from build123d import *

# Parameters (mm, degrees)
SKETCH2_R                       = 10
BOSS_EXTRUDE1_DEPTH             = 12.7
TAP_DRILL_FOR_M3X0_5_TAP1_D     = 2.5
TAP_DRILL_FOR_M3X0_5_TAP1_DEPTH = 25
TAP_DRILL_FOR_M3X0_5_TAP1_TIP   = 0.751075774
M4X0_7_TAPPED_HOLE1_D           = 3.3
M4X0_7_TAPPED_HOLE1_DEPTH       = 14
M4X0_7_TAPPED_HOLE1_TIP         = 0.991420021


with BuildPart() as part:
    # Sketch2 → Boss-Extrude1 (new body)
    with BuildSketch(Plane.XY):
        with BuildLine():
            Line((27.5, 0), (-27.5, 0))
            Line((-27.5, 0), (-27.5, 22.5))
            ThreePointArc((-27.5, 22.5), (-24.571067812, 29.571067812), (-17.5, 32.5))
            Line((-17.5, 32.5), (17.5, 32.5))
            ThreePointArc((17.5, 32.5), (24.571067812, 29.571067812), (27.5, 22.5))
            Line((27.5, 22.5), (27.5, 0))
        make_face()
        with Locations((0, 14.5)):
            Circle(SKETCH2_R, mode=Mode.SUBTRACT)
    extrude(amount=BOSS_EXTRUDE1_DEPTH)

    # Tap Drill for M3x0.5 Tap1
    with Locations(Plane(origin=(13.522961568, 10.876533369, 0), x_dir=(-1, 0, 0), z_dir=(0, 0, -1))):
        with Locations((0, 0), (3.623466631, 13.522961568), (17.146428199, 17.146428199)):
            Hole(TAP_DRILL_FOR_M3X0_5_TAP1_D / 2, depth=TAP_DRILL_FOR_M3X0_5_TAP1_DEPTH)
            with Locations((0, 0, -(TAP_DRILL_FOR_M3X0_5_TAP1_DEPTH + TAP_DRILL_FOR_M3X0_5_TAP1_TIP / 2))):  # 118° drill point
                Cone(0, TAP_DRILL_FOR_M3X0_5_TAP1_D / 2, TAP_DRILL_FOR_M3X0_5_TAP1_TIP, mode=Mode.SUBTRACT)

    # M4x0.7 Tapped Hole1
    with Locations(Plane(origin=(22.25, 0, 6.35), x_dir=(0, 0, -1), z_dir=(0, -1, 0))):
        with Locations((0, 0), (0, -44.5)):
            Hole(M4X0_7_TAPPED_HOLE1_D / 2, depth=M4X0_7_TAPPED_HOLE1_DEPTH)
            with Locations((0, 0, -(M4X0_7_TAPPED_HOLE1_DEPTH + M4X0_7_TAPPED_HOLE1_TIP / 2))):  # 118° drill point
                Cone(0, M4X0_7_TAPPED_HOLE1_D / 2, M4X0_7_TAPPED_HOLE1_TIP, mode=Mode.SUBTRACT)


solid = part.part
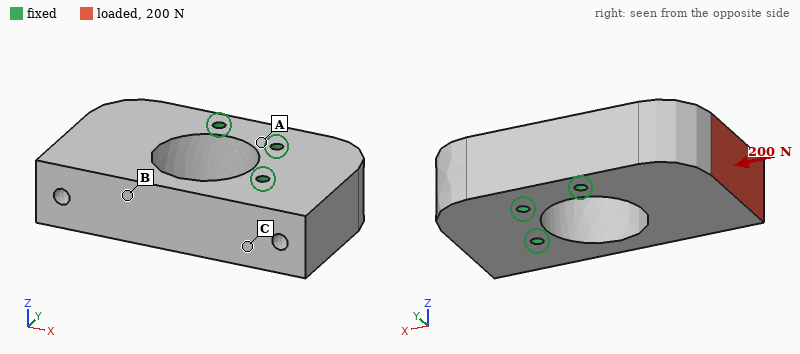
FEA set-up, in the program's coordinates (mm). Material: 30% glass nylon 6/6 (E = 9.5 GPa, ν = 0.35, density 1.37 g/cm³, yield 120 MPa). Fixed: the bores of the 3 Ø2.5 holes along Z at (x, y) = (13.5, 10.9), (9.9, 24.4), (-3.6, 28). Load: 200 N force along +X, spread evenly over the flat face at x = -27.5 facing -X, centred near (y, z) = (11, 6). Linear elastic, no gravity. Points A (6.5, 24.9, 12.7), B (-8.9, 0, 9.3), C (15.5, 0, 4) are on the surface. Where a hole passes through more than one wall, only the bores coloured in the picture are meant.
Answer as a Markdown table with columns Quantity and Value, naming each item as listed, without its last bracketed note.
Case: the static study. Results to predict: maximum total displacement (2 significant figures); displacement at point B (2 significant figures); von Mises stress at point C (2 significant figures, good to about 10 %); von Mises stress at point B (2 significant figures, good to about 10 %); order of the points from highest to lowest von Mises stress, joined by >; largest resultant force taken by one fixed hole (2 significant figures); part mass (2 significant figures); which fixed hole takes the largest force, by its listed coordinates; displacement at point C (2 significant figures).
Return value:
| Quantity | Value |
|---|---|
| maximum total displacement | 13 µm |
| displacement at point B | 8.5 µm |
| von Mises stress at point C | 1.2 MPa |
| von Mises stress at point B | 2.4 MPa |
| order of the points from highest to lowest von Mises stress, joined by > | B > C > A |
| largest resultant force taken by one fixed hole | 160 N |
| part mass | 24 g |
| which fixed hole takes the largest force, by its listed coordinates | (13.5, 10.9) |
| displacement at point C | 3.9 µm |
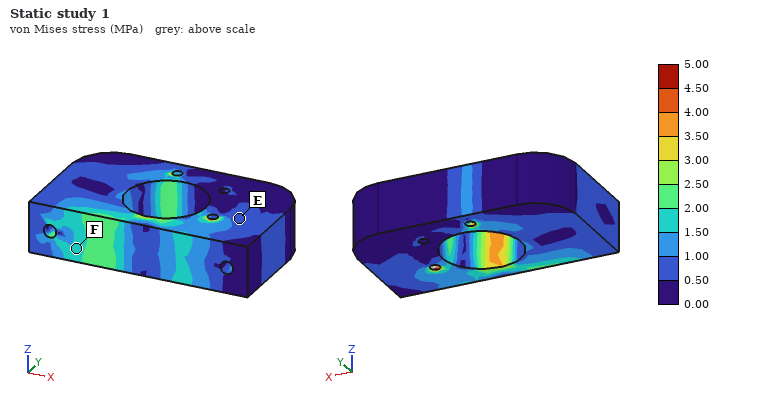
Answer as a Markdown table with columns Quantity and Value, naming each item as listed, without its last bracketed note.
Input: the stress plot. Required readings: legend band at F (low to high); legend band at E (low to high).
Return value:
| Quantity | Value |
|---|---|
| legend band at F | 1.50 to 2.00 MPa |
| legend band at E | 0.50 to 1.00 MPa |
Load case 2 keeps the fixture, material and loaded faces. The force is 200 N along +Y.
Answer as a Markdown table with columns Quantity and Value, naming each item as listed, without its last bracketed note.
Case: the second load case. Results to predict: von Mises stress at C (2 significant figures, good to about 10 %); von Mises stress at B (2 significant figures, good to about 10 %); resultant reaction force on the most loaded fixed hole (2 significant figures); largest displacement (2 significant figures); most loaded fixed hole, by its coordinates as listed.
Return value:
| Quantity | Value |
|---|---|
| von Mises stress at C | 1.8 MPa |
| von Mises stress at B | 2.8 MPa |
| resultant reaction force on the most loaded fixed hole | 290 N |
| largest displacement | 26 µm |
| most loaded fixed hole, by its coordinates as listed | (-3.6, 28) |
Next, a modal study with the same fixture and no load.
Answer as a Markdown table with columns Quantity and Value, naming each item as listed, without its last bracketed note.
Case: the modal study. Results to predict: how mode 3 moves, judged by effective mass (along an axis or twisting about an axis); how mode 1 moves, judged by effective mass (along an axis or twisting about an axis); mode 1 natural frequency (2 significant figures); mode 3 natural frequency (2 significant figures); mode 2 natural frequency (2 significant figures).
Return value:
| Quantity | Value |
|---|---|
| how mode 3 moves, judged by effective mass | twisting about X |
| how mode 1 moves, judged by effective mass | along Z |
| mode 1 natural frequency | 3700 Hz |
| mode 3 natural frequency | 8600 Hz |
| mode 2 natural frequency | 5700 Hz |
